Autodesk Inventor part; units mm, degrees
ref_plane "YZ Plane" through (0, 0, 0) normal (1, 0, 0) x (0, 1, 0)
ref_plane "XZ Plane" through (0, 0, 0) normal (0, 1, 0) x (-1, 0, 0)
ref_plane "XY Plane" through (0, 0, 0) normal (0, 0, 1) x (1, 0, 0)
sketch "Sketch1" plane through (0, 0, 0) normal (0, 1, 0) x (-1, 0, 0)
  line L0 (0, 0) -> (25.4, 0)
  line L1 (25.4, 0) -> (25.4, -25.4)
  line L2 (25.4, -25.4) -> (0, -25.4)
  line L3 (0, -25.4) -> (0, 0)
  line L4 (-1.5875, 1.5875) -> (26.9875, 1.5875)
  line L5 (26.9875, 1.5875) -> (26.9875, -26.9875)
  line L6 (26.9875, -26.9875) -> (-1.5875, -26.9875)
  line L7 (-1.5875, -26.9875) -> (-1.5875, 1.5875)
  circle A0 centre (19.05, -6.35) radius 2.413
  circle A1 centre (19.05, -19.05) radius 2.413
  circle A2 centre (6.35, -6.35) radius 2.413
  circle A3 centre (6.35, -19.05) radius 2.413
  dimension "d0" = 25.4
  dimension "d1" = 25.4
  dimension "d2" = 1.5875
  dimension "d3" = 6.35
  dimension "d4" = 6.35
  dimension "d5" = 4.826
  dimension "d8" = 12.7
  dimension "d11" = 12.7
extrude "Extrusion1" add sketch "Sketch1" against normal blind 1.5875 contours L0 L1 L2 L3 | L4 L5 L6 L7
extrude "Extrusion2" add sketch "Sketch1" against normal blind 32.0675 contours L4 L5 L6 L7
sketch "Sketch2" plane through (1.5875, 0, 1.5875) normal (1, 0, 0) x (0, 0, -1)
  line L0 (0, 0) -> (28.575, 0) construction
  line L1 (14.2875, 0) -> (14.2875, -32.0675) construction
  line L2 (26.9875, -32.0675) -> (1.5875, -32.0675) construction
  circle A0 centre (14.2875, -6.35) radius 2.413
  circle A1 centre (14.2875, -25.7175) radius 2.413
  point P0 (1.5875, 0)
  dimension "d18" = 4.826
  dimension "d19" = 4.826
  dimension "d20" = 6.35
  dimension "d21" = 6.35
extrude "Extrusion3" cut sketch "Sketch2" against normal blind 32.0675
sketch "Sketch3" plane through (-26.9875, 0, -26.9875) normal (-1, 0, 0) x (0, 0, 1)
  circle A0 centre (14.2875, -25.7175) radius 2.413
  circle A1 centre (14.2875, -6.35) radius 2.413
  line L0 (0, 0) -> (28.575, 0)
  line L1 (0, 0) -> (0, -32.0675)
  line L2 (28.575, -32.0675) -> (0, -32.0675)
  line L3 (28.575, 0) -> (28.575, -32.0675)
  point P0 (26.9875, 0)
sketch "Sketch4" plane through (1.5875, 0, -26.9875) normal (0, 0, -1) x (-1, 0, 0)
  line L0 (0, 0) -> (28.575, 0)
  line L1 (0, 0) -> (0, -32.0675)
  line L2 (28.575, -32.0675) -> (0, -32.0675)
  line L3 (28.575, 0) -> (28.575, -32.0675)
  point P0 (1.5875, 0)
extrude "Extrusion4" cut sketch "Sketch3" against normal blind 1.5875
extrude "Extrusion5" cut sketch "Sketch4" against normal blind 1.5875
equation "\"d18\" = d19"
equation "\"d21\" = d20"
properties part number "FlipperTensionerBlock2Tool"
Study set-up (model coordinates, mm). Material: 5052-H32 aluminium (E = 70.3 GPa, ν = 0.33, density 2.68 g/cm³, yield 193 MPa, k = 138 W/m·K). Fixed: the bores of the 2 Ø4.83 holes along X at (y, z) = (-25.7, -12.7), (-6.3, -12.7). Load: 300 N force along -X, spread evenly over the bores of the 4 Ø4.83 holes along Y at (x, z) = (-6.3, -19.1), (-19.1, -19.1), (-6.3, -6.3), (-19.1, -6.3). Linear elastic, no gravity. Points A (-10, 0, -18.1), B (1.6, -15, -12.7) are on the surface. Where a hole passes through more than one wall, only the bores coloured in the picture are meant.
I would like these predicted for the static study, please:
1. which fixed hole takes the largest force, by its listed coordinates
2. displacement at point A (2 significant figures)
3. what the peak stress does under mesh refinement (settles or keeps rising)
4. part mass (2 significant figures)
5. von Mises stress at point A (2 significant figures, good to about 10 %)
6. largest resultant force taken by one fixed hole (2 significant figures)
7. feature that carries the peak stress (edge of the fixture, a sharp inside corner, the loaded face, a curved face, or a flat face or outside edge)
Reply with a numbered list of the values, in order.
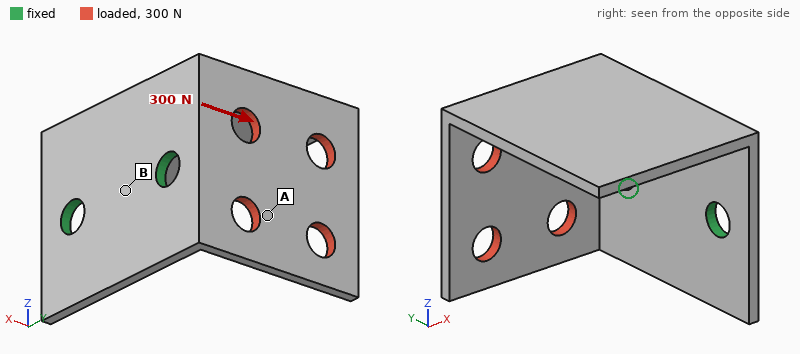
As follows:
1. (-6.3, -12.7)
2. 39 µm
3. keeps rising
4. 9.4 g
5. 16 MPa
6. 320 N
7. edge of the fixture
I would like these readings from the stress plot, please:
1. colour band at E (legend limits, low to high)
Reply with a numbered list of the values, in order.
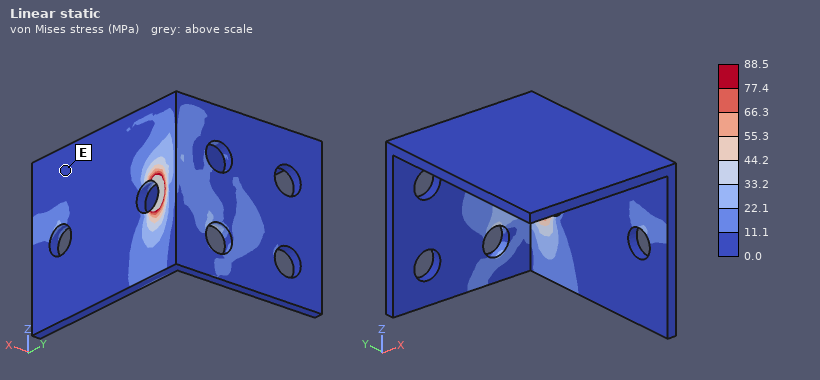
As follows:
1. 0.0 to 11.1 MPa
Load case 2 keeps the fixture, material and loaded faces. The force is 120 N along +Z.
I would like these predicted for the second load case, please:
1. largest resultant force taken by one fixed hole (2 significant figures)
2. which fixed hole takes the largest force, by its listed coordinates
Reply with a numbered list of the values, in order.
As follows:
1. 140 N
2. (-6.3, -12.7)
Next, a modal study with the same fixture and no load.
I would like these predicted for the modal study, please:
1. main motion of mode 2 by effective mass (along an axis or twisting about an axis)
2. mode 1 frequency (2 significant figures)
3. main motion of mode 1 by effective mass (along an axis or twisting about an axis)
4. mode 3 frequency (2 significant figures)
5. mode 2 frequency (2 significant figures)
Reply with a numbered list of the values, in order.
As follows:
1. along Y
2. 1800 Hz
3. along Z
4. 3500 Hz
5. 2300 Hz
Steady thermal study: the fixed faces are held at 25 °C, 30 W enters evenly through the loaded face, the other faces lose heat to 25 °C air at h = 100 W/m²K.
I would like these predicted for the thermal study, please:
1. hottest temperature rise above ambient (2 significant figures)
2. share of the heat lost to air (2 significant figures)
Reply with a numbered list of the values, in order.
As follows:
1. 70 K
2. 36 %
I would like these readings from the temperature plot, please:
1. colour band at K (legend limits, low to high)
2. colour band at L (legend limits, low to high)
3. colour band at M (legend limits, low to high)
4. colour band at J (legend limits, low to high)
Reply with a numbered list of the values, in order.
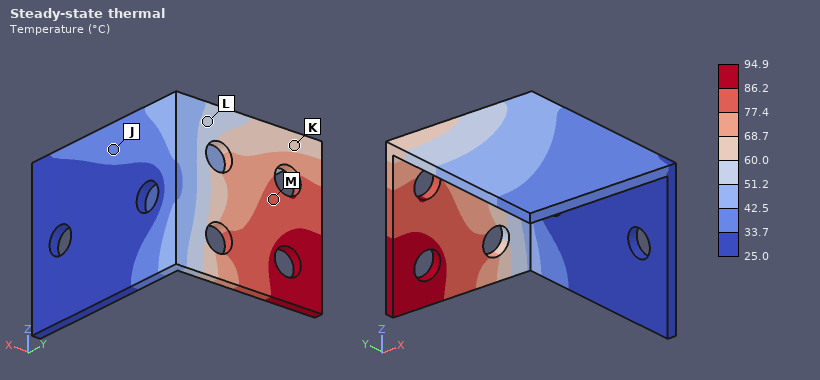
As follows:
1. 60.0 to 68.7 °C
2. 51.2 to 60.0 °C
3. 77.4 to 86.2 °C
4. 33.7 to 42.5 °C
